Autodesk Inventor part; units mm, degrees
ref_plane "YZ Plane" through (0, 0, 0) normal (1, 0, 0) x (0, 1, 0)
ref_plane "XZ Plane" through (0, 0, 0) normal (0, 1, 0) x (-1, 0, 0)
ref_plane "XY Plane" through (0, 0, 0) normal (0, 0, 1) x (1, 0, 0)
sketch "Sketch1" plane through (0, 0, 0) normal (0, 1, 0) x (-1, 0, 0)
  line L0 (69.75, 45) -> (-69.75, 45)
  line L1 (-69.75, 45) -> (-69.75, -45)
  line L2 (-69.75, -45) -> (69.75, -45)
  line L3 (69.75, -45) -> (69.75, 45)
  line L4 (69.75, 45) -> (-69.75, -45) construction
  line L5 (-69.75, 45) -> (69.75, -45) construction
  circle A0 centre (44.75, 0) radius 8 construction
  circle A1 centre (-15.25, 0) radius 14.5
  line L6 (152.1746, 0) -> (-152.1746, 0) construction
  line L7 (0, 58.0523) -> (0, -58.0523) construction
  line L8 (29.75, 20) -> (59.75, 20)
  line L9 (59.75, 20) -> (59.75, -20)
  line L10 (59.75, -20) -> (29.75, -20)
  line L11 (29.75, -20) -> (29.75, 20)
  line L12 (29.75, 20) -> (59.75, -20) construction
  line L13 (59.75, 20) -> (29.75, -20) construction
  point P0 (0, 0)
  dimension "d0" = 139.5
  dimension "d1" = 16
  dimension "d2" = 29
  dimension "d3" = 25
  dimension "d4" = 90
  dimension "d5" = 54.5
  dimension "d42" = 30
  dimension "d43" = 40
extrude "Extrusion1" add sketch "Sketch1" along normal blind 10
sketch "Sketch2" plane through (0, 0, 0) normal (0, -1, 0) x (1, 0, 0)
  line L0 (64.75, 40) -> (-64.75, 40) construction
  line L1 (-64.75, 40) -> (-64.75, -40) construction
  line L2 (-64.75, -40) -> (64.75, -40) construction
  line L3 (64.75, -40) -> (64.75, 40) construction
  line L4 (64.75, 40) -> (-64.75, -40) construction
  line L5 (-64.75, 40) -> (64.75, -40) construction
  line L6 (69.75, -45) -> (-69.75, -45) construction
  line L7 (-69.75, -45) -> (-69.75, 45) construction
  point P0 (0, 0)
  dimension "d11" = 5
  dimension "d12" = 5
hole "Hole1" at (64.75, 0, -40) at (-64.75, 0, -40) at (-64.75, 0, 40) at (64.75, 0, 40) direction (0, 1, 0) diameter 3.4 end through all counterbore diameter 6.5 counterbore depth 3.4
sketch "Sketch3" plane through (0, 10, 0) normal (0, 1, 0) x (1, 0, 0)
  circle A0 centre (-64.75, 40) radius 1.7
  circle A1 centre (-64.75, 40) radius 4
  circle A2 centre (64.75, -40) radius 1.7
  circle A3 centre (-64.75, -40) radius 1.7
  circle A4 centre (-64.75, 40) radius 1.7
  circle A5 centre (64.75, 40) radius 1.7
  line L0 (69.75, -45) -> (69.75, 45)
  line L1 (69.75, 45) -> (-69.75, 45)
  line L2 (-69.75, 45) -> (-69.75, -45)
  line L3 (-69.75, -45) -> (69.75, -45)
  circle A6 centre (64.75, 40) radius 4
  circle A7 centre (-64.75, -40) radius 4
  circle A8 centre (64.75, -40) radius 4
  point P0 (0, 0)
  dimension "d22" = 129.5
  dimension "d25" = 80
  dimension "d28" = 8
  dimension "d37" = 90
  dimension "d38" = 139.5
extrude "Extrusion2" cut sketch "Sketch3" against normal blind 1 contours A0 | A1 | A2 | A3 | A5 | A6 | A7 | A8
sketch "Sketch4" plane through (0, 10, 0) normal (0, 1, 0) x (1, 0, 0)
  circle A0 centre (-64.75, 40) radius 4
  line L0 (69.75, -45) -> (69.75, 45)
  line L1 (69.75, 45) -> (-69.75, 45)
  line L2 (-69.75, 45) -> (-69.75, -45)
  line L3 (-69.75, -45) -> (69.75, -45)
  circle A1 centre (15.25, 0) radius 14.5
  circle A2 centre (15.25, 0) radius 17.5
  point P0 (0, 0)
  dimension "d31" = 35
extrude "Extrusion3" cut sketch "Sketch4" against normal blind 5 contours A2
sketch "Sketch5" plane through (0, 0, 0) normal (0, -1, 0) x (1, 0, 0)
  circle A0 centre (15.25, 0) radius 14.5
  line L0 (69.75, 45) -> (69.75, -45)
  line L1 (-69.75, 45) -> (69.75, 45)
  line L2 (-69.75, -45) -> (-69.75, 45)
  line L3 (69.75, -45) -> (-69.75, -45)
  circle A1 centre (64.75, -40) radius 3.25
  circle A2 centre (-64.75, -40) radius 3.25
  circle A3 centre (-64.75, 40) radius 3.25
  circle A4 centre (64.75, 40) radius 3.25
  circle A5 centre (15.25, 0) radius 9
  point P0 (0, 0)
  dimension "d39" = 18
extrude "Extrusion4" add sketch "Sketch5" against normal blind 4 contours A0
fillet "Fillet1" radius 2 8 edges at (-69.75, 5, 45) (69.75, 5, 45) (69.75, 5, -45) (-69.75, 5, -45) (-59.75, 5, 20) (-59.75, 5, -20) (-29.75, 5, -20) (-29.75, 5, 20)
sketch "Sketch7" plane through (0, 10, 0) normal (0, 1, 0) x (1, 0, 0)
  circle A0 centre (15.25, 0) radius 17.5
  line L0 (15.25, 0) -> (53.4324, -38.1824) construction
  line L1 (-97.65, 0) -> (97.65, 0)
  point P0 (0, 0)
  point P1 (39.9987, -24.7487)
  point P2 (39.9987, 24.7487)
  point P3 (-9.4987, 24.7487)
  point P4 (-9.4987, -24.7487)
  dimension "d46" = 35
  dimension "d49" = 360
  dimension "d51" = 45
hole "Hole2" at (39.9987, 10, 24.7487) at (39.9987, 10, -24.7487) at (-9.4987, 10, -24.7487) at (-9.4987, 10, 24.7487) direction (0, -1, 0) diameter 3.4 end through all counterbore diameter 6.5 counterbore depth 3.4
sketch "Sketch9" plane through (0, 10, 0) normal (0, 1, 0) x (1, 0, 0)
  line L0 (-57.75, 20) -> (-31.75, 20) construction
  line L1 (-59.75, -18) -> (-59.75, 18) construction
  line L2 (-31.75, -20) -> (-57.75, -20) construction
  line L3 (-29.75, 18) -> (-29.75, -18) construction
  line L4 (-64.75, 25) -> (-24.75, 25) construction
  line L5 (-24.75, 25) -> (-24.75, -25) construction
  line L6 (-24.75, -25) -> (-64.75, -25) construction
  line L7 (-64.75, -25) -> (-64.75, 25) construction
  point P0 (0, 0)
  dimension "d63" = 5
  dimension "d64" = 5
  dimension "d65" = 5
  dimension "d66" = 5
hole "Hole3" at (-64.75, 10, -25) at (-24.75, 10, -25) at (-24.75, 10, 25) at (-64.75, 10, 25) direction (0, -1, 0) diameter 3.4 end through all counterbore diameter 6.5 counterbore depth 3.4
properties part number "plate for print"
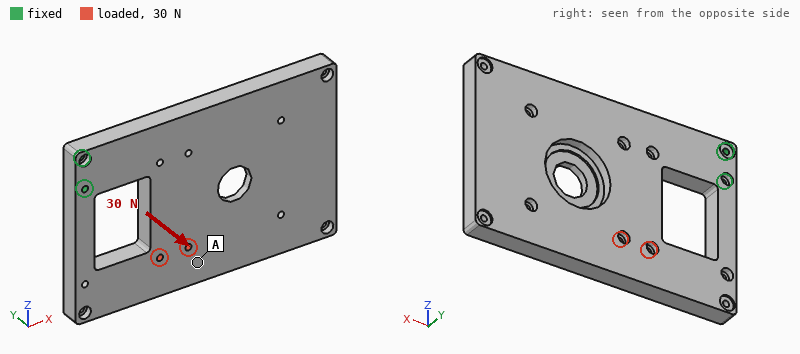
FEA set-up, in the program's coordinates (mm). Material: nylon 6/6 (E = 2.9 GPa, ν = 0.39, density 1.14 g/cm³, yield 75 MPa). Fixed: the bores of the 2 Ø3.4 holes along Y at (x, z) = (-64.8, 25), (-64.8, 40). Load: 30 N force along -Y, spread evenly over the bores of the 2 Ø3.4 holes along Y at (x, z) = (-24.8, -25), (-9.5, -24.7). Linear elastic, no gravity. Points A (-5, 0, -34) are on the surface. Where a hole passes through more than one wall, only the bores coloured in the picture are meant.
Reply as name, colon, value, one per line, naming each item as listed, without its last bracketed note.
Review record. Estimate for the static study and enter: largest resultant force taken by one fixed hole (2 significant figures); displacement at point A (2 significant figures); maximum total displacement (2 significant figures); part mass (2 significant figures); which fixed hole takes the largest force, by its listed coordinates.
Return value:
largest resultant force taken by one fixed hole: 96 N
displacement at point A: 0.91 mm
maximum total displacement: 1.6 mm
part mass: 120 g
which fixed hole takes the largest force, by its listed coordinates: (-64.8, 25)
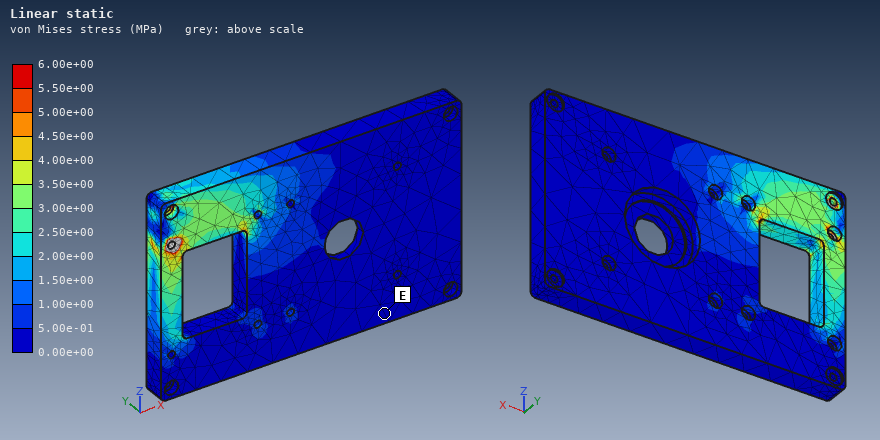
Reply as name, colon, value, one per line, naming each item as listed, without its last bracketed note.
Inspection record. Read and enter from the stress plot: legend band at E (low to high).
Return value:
legend band at E: 0.00e+00 to 5.00e-01 MPa
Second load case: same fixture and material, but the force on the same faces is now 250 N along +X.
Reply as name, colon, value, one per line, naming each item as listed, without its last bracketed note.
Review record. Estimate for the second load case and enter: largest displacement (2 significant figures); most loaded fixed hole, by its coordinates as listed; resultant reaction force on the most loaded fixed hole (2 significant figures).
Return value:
largest displacement: 1.8 mm
most loaded fixed hole, by its coordinates as listed: (-64.8, 25)
resultant reaction force on the most loaded fixed hole: 940 N
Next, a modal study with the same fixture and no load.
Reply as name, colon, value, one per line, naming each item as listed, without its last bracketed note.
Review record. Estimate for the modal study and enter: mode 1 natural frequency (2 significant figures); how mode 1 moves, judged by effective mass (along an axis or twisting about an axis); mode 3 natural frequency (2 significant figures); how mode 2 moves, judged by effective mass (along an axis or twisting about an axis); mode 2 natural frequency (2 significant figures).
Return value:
mode 1 natural frequency: 72 Hz
how mode 1 moves, judged by effective mass: along Y
mode 3 natural frequency: 220 Hz
how mode 2 moves, judged by effective mass: along Z
mode 2 natural frequency: 190 Hz
